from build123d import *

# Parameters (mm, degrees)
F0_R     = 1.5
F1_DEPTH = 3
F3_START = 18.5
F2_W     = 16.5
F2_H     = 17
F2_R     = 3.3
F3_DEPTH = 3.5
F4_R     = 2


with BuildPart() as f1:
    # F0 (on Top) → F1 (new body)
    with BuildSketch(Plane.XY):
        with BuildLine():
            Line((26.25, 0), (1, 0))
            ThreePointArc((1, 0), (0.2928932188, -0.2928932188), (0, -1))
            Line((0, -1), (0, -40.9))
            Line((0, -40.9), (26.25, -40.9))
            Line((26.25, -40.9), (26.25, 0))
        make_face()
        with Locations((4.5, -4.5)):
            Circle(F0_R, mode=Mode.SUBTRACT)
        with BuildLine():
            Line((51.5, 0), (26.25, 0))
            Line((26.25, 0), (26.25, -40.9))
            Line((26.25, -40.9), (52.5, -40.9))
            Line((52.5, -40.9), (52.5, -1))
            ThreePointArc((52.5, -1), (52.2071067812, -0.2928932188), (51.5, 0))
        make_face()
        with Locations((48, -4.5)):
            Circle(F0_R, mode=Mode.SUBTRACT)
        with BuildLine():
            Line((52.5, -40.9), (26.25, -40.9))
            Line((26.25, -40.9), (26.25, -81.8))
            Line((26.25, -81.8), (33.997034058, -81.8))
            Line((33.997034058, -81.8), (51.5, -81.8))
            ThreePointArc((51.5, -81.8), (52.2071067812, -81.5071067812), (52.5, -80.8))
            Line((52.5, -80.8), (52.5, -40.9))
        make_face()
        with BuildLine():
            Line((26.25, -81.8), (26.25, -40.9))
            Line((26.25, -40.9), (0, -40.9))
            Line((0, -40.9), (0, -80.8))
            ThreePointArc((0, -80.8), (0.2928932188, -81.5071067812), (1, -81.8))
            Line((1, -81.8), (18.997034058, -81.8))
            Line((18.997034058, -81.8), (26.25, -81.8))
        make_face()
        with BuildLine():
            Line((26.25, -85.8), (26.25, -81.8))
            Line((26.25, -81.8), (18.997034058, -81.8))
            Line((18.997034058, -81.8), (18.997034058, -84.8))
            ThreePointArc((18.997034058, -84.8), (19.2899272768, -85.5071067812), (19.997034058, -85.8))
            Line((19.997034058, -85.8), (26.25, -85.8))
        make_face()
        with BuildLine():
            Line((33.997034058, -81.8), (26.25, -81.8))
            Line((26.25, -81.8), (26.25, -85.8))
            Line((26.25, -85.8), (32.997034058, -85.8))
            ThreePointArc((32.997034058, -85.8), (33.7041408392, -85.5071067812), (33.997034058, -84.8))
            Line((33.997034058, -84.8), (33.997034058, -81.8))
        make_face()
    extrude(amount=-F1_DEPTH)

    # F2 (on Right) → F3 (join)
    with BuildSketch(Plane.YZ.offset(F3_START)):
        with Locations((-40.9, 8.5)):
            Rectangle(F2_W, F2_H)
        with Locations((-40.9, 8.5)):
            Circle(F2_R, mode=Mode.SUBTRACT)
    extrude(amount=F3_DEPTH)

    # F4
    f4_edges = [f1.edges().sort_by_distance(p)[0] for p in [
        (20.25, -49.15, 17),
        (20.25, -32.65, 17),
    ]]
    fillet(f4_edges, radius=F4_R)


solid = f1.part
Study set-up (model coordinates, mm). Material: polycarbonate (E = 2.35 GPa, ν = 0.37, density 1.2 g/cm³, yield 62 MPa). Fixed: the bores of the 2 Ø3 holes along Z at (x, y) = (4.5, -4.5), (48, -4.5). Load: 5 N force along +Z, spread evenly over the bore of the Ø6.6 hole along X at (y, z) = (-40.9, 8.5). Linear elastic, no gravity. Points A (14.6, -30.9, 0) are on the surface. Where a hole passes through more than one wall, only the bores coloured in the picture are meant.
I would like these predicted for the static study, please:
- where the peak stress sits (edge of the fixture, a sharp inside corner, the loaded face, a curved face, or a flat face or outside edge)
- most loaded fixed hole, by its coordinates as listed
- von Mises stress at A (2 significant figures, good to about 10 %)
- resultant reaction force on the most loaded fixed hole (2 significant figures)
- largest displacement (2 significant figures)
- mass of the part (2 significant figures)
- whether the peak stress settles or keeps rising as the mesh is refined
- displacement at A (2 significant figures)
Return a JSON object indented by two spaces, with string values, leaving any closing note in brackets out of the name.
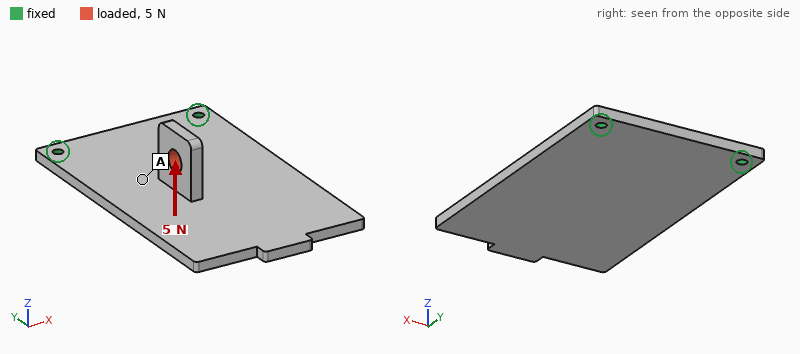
{
  "where the peak stress sits": "edge of the fixture",
  "most loaded fixed hole, by its coordinates as listed": "(4.5, -4.5)",
  "von Mises stress at A": "0.75 MPa",
  "resultant reaction force on the most loaded fixed hole": "3.2 N",
  "largest displacement": "1.1 mm",
  "mass of the part": "17 g",
  "whether the peak stress settles or keeps rising as the mesh is refined": "keeps rising",
  "displacement at A": "0.28 mm"
}
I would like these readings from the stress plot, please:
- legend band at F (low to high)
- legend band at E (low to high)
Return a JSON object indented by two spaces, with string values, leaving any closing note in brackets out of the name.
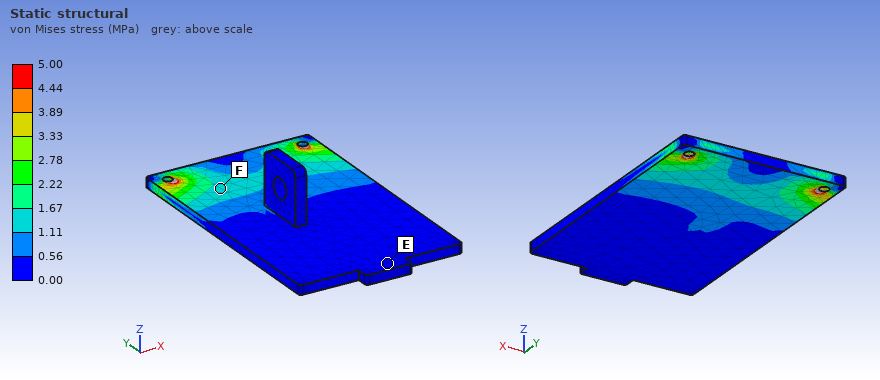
{
  "legend band at F": "1.11 to 1.67 MPa",
  "legend band at E": "0.00 to 0.56 MPa"
}
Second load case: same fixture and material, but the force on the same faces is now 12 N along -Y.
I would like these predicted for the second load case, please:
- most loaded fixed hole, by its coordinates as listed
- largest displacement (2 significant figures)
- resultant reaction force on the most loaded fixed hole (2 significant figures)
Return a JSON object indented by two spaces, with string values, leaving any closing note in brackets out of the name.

{
  "most loaded fixed hole, by its coordinates as listed": "(4.5, -4.5)",
  "largest displacement": "1.1 mm",
  "resultant reaction force on the most loaded fixed hole": "7.9 N"
}
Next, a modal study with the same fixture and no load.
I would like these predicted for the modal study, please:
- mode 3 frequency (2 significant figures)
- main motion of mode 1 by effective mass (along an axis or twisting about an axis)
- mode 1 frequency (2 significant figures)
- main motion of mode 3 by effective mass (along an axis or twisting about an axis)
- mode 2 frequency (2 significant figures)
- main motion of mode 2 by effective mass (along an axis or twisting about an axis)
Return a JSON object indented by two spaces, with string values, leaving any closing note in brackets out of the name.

{
  "mode 3 frequency": "640 Hz",
  "main motion of mode 1 by effective mass": "along Z",
  "mode 1 frequency": "98 Hz",
  "main motion of mode 3 by effective mass": "along Z",
  "mode 2 frequency": "370 Hz",
  "main motion of mode 2 by effective mass": "twisting about Y"
}
